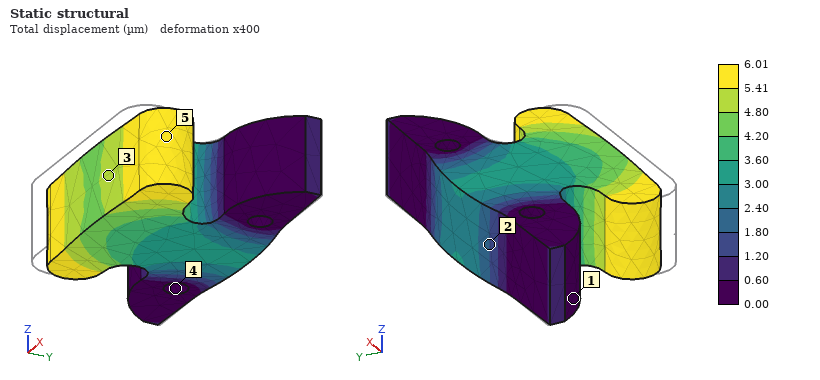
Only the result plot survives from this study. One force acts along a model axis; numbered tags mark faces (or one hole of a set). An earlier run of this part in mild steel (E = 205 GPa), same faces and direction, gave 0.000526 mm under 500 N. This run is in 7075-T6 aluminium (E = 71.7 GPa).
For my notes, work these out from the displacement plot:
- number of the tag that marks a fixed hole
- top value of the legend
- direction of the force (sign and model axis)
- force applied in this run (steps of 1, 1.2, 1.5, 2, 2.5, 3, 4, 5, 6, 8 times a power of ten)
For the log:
4
6.01 µm
+Y
2 kN
